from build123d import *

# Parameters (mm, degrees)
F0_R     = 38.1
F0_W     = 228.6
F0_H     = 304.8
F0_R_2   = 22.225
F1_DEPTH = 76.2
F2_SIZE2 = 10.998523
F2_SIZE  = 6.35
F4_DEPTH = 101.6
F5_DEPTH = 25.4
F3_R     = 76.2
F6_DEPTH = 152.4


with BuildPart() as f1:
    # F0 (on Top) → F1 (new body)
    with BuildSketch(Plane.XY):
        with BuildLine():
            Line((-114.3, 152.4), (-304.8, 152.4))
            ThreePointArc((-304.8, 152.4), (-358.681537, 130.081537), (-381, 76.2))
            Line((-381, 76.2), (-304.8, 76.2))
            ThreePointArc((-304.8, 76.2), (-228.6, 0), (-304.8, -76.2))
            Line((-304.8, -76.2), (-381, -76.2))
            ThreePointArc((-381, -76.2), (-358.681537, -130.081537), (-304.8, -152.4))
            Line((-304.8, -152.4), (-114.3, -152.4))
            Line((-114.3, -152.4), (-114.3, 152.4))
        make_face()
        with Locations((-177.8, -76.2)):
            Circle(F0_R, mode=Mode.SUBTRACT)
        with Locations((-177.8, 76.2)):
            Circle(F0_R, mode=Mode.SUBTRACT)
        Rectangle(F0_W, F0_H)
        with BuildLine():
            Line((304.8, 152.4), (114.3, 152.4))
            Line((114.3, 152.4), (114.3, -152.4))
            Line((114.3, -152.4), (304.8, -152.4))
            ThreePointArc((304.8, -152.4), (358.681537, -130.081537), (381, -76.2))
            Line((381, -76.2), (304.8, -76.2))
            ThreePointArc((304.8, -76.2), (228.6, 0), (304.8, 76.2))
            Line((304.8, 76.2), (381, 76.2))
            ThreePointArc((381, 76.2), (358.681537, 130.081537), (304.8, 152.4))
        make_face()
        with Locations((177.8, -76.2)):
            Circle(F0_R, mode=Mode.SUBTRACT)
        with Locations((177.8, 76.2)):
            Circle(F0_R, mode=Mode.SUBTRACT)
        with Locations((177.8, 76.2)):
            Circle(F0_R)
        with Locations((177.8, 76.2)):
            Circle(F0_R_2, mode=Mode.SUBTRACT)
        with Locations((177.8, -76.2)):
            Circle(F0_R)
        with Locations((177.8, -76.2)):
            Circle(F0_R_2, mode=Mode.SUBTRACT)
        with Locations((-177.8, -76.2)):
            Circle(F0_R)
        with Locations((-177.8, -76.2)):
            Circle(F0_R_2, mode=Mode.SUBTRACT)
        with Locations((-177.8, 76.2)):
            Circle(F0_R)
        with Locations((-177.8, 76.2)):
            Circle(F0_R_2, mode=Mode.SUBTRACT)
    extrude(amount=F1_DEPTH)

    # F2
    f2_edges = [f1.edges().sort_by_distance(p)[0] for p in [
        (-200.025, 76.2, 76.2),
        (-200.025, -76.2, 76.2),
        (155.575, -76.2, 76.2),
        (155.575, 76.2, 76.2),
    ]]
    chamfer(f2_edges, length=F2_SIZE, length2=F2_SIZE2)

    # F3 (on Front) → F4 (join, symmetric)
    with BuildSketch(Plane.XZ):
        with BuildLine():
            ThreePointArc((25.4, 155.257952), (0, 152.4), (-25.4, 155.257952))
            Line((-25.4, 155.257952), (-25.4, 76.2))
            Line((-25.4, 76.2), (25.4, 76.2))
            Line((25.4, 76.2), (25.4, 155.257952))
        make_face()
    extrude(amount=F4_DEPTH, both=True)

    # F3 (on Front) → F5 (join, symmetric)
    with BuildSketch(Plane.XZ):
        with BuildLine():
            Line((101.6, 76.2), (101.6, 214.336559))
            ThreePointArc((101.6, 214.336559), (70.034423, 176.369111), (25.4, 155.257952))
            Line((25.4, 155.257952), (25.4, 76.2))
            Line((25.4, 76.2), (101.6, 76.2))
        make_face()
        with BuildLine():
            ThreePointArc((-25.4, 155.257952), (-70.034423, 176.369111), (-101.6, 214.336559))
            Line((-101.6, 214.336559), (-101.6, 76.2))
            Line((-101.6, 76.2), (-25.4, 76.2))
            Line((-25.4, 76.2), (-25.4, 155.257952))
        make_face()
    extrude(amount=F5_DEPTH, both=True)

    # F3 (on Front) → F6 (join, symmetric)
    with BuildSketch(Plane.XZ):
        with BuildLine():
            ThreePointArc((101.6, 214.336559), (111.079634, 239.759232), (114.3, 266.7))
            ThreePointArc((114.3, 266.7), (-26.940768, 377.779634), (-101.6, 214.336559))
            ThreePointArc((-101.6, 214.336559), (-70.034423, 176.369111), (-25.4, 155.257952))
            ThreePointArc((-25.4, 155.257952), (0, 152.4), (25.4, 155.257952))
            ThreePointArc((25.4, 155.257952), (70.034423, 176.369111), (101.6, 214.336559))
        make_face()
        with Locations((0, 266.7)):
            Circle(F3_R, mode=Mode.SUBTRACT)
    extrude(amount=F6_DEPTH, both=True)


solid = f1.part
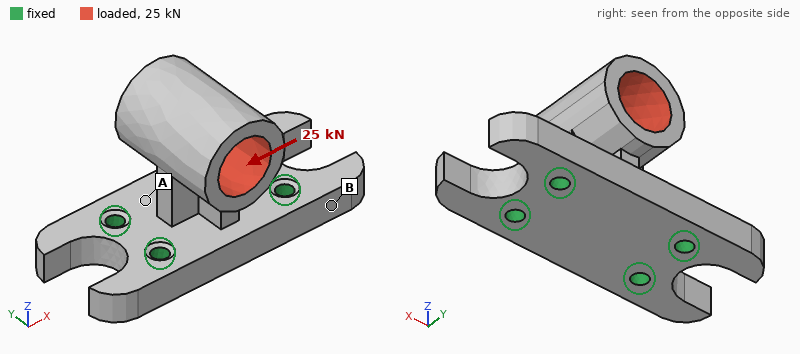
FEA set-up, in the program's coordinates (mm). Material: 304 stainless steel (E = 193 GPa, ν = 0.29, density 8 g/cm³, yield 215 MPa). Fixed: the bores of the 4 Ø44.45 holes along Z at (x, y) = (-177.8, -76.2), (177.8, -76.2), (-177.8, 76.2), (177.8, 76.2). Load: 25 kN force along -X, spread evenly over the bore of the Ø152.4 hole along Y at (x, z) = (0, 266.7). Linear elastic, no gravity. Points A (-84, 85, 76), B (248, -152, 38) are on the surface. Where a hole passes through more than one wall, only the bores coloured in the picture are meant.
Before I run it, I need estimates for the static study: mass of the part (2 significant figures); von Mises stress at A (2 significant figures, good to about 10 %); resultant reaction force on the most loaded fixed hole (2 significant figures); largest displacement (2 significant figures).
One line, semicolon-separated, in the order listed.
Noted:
180 kg; 2.3 MPa; 12 kN; 43 µm
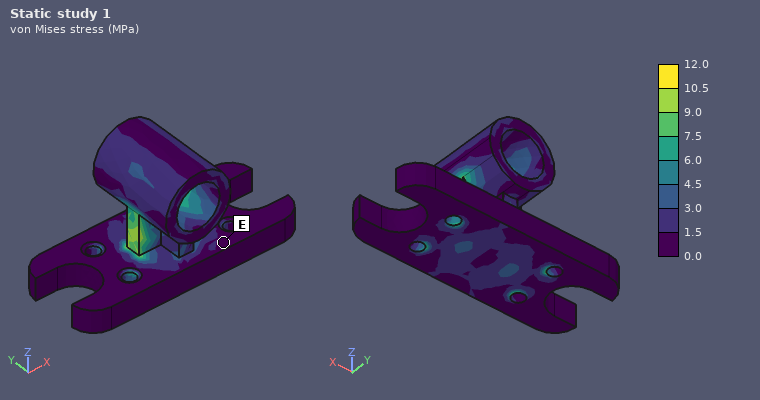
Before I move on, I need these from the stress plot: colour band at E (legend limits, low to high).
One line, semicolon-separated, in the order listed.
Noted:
0.0 to 1.5 MPa
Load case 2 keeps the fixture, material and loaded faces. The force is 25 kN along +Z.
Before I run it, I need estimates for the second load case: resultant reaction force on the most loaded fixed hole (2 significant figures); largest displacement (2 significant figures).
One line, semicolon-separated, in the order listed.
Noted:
6.5 kN; 6.6 µm
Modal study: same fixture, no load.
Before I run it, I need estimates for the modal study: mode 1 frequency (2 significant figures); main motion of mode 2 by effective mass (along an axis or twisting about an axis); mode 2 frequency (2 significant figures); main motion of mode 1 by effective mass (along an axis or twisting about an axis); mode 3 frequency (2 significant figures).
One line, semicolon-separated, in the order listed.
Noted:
500 Hz; along X; 570 Hz; along Y; 870 Hz
